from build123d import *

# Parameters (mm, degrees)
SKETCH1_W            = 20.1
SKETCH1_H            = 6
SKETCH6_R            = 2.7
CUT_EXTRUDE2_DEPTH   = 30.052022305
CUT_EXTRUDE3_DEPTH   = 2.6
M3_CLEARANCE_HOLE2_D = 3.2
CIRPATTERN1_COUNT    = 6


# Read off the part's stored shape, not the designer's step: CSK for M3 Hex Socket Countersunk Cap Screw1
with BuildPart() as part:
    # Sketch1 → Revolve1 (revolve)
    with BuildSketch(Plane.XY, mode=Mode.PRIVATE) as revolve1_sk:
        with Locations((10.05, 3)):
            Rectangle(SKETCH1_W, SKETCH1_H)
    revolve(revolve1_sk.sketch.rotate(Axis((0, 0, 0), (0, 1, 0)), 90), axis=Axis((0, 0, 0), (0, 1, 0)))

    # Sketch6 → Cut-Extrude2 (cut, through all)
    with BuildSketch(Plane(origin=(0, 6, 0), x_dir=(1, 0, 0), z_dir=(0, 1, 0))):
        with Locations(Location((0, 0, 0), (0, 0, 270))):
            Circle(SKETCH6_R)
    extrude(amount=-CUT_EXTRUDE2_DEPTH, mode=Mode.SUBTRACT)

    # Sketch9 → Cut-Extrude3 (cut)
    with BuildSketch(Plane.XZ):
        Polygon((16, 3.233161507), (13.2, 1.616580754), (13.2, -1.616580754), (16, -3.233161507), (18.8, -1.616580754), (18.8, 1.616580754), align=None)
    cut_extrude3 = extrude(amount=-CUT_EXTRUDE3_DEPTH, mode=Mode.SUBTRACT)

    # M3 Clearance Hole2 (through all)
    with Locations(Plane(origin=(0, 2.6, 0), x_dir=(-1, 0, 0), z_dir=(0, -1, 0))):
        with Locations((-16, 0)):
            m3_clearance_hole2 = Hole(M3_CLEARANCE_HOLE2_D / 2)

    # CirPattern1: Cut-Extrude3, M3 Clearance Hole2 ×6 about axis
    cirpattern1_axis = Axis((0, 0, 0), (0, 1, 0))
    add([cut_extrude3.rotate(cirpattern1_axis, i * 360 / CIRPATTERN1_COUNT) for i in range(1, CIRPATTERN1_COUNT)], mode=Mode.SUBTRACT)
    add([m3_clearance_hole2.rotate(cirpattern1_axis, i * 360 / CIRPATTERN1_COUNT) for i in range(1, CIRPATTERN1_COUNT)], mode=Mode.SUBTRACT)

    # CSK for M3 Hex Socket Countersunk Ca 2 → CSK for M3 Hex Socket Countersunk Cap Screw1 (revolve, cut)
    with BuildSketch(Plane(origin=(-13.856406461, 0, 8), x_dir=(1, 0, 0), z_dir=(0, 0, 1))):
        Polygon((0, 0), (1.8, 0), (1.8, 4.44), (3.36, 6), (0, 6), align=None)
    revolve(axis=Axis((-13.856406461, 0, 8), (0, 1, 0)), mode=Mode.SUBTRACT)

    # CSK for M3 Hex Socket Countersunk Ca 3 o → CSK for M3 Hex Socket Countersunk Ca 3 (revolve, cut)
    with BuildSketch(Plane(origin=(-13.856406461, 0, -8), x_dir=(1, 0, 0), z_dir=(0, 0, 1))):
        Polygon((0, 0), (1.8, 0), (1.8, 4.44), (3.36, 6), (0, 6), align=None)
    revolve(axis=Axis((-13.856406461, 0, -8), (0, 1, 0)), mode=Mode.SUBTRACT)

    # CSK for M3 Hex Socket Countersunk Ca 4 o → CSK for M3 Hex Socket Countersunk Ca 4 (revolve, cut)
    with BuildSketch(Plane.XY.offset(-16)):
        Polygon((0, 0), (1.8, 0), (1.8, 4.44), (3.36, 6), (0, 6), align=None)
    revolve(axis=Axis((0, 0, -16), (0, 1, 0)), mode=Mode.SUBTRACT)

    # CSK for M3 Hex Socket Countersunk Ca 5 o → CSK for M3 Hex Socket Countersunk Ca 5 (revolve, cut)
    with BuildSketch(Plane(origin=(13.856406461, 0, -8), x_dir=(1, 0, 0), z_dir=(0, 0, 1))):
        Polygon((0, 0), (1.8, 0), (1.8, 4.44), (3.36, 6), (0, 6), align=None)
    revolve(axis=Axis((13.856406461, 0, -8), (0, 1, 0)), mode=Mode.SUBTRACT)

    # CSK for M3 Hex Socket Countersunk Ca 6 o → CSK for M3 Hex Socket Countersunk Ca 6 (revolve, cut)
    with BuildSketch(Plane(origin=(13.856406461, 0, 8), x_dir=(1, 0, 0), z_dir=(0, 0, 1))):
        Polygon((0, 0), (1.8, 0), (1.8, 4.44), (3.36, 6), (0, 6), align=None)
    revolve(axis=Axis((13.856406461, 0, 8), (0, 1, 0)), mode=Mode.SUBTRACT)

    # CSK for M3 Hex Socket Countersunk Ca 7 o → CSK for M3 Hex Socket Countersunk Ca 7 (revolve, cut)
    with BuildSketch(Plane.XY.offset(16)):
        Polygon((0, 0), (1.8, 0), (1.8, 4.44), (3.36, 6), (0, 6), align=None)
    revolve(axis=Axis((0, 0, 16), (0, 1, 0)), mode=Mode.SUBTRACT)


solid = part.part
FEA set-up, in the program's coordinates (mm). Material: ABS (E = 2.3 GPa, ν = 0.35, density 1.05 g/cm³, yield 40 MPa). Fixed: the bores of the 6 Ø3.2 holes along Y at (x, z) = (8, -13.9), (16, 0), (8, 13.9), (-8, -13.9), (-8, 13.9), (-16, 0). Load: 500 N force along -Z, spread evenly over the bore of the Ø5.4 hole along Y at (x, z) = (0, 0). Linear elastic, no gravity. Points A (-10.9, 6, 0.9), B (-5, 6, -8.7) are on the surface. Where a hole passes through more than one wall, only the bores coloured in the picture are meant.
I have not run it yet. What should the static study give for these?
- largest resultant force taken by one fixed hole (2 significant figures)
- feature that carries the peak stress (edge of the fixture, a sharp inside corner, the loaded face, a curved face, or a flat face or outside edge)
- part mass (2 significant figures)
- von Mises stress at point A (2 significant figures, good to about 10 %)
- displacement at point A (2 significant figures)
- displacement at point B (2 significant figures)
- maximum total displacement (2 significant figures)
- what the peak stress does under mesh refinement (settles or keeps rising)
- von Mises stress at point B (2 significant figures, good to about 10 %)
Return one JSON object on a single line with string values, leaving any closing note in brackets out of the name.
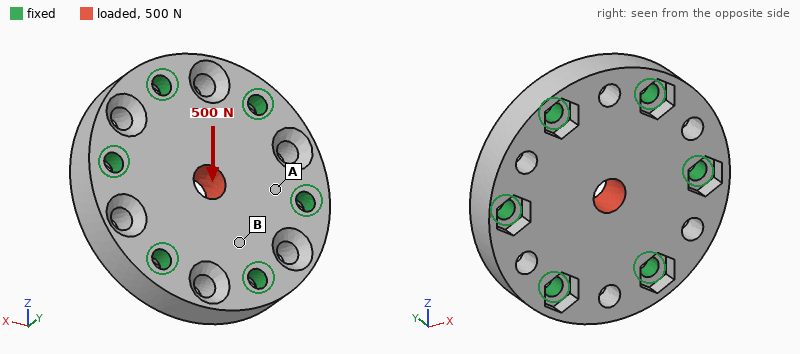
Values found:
{"largest resultant force taken by one fixed hole": "110 N", "feature that carries the peak stress": "edge of the fixture", "part mass": "6.7 g", "von Mises stress at point A": "0.84 MPa", "displacement at point A": "5.1 µm", "displacement at point B": "8.0 µm", "maximum total displacement": "23 µm", "what the peak stress does under mesh refinement": "keeps rising", "von Mises stress at point B": "3.7 MPa"}
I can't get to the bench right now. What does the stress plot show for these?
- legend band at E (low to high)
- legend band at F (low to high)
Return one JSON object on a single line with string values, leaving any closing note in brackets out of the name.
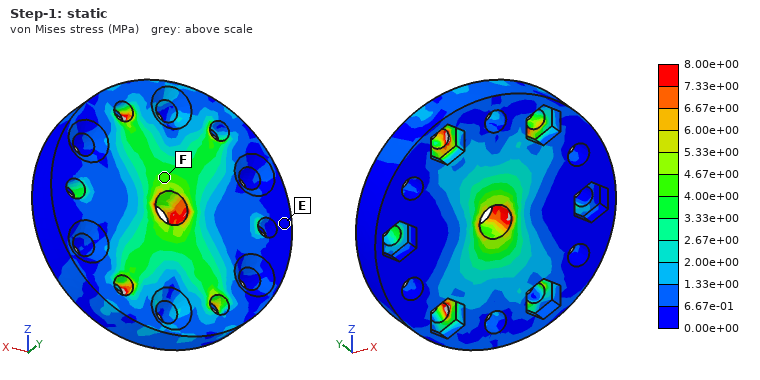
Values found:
{"legend band at E": "0.00e+00 to 6.67e-01 MPa", "legend band at F": "4.00e+00 to 4.67e+00 MPa"}
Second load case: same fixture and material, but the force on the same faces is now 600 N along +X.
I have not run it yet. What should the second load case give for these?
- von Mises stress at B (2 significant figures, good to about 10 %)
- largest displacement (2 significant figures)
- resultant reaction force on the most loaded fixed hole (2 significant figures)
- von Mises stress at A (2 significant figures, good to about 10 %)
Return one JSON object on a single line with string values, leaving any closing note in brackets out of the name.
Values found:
{"von Mises stress at B": "2.7 MPa", "largest displacement": "27 µm", "resultant reaction force on the most loaded fixed hole": "150 N", "von Mises stress at A": "5.0 MPa"}
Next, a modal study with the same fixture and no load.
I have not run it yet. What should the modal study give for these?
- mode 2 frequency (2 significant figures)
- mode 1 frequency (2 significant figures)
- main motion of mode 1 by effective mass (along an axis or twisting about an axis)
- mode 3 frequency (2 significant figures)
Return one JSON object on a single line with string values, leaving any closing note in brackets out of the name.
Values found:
{"mode 2 frequency": "16 kHz", "mode 1 frequency": "9800 Hz", "main motion of mode 1 by effective mass": "along Y", "mode 3 frequency": "16 kHz"}
